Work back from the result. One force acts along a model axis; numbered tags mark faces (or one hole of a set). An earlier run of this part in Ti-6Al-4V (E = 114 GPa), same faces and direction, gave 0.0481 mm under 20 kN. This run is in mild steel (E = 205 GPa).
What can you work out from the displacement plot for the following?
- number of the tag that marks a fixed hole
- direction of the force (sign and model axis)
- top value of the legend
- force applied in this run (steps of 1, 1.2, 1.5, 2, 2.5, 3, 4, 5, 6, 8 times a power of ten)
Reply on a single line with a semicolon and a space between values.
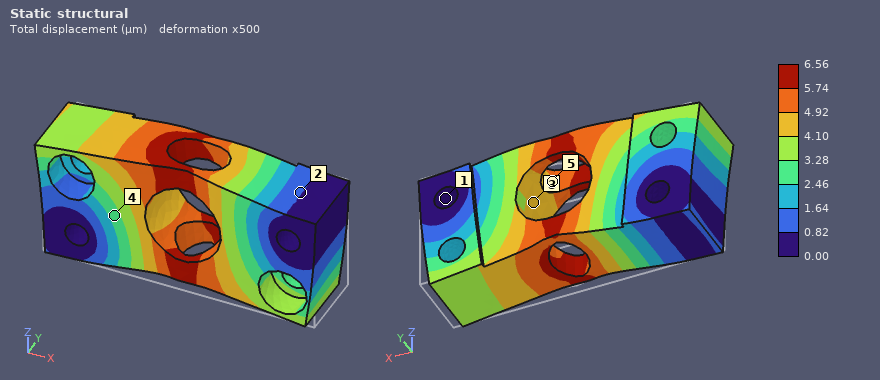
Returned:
1; +Z; 6.56 µm; 5 kN
